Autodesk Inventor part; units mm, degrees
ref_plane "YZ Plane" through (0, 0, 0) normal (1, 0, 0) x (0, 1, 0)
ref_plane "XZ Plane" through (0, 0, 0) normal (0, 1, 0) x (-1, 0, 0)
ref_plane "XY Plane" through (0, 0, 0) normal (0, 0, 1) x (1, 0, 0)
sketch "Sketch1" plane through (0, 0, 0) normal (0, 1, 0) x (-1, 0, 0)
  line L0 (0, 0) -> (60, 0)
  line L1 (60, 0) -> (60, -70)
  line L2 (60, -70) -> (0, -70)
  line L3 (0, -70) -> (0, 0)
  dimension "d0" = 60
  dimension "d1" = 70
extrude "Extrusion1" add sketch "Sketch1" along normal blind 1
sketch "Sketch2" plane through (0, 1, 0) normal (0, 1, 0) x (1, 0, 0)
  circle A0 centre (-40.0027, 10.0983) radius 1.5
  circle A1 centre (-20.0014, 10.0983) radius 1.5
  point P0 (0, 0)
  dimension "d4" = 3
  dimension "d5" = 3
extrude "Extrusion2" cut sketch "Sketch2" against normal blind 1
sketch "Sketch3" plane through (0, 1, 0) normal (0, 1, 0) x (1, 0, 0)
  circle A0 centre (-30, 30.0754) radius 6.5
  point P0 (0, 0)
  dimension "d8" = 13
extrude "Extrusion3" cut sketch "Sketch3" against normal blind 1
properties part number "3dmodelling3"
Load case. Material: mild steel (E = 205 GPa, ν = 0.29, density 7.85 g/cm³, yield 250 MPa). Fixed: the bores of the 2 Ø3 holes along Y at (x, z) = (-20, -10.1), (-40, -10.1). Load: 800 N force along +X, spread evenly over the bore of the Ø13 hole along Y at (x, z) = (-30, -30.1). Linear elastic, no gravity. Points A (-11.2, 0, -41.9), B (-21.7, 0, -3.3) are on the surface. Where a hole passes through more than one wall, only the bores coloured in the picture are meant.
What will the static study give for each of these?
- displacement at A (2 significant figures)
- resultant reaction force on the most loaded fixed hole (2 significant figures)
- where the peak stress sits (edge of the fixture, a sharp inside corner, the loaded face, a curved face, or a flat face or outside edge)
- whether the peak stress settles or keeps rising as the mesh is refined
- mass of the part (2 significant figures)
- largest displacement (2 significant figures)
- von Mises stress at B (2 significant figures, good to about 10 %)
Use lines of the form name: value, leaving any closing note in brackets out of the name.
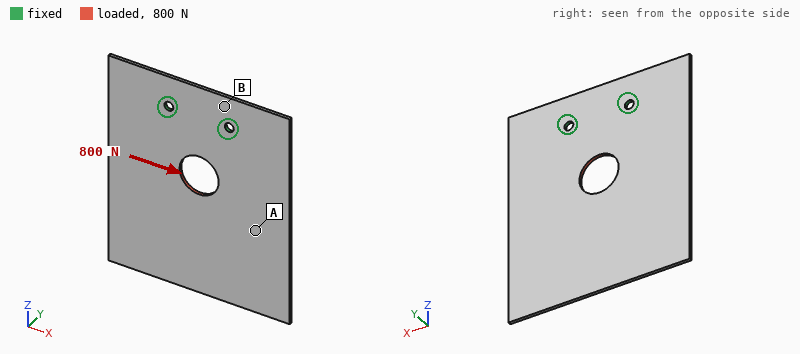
displacement at A: 19 µm
resultant reaction force on the most loaded fixed hole: 820 N
where the peak stress sits: edge of the fixture
whether the peak stress settles or keeps rising as the mesh is refined: keeps rising
mass of the part: 32 g
largest displacement: 29 µm
von Mises stress at B: 28 MPa
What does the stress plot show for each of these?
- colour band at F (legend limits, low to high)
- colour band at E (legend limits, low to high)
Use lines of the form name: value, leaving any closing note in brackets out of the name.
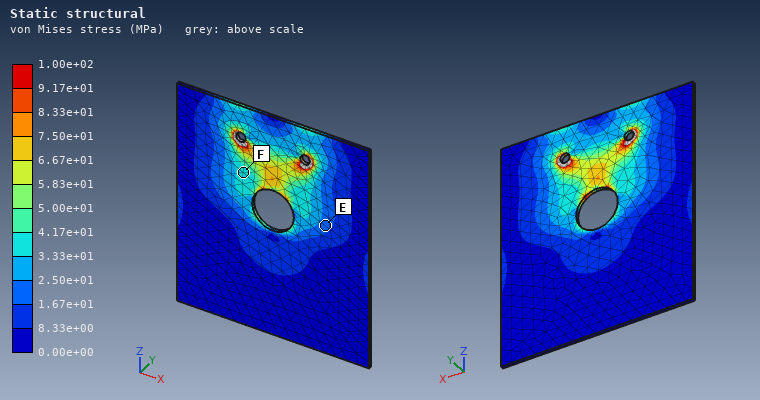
colour band at F: 3.33e+01 to 4.17e+01 MPa
colour band at E: 1.67e+01 to 2.50e+01 MPa
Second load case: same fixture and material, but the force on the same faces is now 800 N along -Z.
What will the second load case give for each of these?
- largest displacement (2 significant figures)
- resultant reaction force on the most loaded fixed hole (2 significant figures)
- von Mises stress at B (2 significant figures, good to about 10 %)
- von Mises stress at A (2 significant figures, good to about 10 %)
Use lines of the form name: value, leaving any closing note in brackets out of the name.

largest displacement: 4.0 µm
resultant reaction force on the most loaded fixed hole: 400 N
von Mises stress at B: 10.0 MPa
von Mises stress at A: 5.4 MPa
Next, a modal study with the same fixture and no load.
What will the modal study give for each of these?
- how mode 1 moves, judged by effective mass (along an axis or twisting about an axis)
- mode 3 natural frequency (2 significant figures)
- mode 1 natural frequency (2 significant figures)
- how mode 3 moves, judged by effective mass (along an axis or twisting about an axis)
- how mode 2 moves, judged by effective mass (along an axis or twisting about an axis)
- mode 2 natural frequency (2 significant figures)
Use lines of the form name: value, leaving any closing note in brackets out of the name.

how mode 1 moves, judged by effective mass: along Y
mode 3 natural frequency: 1200 Hz
mode 1 natural frequency: 210 Hz
how mode 3 moves, judged by effective mass: along Y
how mode 2 moves, judged by effective mass: twisting about Z
mode 2 natural frequency: 490 Hz
